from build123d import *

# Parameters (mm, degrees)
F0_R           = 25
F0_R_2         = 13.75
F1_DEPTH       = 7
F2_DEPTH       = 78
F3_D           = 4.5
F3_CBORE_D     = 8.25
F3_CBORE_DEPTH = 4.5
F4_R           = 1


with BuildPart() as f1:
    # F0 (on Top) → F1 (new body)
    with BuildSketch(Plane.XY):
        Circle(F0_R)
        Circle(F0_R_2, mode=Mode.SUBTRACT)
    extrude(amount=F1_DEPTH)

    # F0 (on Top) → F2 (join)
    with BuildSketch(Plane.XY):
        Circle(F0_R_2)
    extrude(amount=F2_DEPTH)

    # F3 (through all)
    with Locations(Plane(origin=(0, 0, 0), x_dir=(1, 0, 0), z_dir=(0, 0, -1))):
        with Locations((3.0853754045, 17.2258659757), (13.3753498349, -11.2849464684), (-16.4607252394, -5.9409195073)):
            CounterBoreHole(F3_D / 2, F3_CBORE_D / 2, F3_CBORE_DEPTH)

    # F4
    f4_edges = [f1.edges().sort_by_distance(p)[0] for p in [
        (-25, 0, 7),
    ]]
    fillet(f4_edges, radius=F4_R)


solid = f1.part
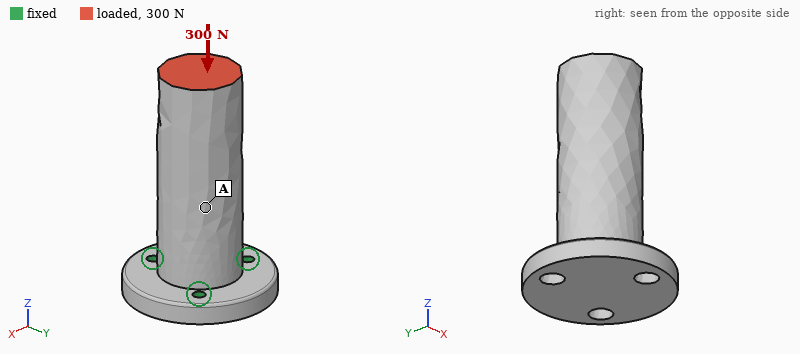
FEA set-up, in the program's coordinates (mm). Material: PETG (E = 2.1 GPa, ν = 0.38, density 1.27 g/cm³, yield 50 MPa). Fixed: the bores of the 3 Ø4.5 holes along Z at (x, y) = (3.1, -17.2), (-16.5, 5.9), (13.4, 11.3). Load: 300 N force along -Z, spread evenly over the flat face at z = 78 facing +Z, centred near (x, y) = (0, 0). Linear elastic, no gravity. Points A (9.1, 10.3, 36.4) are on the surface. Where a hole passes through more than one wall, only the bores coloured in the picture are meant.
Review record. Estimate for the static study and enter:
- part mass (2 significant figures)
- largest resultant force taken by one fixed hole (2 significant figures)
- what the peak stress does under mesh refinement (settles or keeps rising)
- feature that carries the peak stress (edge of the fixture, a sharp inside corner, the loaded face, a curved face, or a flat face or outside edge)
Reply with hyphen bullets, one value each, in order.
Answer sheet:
- 70 g
- 100 N
- keeps rising
- edge of the fixture
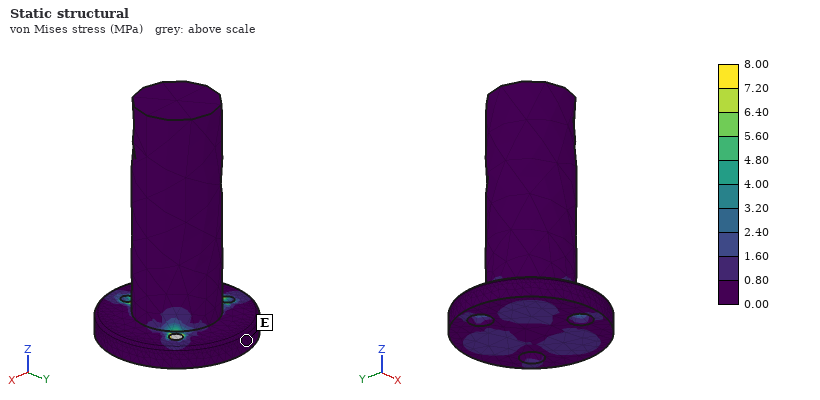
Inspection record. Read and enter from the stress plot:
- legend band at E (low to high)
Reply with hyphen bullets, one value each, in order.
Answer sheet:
- 0.00 to 0.80 MPa
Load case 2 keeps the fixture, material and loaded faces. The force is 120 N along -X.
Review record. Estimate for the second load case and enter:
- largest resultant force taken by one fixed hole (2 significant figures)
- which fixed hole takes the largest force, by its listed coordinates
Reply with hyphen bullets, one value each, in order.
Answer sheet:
- 310 N
- (-16.5, 5.9)
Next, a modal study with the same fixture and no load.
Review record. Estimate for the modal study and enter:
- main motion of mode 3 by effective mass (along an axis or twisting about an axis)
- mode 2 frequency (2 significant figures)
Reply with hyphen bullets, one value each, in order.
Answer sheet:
- along Z
- 570 Hz
